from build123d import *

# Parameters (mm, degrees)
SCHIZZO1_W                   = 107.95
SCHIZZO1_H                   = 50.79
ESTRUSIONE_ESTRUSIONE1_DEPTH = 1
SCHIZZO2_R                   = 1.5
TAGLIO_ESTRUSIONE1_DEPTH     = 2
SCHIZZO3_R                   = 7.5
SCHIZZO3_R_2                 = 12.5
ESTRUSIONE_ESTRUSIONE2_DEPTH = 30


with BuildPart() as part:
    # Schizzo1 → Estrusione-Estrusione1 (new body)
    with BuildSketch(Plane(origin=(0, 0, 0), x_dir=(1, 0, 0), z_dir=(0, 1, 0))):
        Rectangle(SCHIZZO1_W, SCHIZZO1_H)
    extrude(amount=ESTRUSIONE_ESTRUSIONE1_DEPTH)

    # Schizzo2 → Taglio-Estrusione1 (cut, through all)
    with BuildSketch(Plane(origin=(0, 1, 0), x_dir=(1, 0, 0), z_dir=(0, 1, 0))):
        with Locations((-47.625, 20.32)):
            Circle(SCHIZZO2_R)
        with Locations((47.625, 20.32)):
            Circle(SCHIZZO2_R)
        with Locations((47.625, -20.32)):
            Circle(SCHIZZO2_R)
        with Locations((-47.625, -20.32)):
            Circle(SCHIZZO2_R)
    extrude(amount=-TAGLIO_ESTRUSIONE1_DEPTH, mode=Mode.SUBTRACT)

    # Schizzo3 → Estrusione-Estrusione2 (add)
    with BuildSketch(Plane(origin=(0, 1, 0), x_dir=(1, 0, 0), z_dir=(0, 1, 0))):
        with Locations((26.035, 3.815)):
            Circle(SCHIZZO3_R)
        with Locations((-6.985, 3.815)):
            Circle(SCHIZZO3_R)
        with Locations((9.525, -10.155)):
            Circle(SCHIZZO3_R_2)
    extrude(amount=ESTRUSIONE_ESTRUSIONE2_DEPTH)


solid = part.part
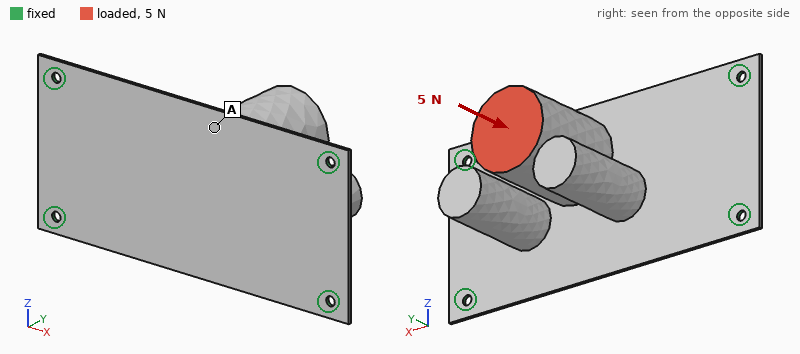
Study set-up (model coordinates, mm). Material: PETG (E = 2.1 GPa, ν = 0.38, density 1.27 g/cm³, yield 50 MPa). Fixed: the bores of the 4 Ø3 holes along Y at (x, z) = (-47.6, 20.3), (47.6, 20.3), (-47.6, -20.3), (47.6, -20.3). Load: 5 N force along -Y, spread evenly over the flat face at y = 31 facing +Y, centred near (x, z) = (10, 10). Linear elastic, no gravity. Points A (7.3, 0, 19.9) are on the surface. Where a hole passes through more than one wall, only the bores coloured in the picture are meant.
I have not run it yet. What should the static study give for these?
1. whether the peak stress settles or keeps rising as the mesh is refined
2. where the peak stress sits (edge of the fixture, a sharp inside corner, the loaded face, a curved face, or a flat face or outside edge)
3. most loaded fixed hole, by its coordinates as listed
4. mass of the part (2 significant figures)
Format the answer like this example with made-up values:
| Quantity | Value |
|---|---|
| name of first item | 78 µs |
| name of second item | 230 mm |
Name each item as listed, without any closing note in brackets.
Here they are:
| Quantity | Value |
|---|---|
| whether the peak stress settles or keeps rising as the mesh is refined | keeps rising |
| where the peak stress sits | edge of the fixture |
| most loaded fixed hole, by its coordinates as listed | (47.6, 20.3) |
| mass of the part | 39 g |
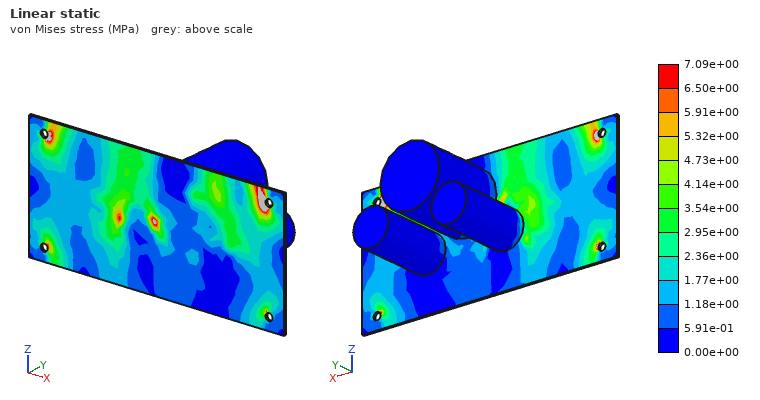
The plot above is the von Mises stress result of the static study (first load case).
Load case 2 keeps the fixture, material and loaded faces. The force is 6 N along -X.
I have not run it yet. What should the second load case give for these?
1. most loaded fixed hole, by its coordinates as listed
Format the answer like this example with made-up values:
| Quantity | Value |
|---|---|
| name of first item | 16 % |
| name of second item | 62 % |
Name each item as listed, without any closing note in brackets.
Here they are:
| Quantity | Value |
|---|---|
| most loaded fixed hole, by its coordinates as listed | (-47.6, -20.3) |
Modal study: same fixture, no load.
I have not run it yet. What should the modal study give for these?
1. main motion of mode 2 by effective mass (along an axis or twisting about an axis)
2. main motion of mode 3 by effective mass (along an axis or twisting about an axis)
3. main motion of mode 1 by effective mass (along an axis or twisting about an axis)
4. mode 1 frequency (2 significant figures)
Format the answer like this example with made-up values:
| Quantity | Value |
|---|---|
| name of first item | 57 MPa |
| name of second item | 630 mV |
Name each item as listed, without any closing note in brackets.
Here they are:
| Quantity | Value |
|---|---|
| main motion of mode 2 by effective mass | along Z |
| main motion of mode 3 by effective mass | along X |
| main motion of mode 1 by effective mass | along Y |
| mode 1 frequency | 60 Hz |
